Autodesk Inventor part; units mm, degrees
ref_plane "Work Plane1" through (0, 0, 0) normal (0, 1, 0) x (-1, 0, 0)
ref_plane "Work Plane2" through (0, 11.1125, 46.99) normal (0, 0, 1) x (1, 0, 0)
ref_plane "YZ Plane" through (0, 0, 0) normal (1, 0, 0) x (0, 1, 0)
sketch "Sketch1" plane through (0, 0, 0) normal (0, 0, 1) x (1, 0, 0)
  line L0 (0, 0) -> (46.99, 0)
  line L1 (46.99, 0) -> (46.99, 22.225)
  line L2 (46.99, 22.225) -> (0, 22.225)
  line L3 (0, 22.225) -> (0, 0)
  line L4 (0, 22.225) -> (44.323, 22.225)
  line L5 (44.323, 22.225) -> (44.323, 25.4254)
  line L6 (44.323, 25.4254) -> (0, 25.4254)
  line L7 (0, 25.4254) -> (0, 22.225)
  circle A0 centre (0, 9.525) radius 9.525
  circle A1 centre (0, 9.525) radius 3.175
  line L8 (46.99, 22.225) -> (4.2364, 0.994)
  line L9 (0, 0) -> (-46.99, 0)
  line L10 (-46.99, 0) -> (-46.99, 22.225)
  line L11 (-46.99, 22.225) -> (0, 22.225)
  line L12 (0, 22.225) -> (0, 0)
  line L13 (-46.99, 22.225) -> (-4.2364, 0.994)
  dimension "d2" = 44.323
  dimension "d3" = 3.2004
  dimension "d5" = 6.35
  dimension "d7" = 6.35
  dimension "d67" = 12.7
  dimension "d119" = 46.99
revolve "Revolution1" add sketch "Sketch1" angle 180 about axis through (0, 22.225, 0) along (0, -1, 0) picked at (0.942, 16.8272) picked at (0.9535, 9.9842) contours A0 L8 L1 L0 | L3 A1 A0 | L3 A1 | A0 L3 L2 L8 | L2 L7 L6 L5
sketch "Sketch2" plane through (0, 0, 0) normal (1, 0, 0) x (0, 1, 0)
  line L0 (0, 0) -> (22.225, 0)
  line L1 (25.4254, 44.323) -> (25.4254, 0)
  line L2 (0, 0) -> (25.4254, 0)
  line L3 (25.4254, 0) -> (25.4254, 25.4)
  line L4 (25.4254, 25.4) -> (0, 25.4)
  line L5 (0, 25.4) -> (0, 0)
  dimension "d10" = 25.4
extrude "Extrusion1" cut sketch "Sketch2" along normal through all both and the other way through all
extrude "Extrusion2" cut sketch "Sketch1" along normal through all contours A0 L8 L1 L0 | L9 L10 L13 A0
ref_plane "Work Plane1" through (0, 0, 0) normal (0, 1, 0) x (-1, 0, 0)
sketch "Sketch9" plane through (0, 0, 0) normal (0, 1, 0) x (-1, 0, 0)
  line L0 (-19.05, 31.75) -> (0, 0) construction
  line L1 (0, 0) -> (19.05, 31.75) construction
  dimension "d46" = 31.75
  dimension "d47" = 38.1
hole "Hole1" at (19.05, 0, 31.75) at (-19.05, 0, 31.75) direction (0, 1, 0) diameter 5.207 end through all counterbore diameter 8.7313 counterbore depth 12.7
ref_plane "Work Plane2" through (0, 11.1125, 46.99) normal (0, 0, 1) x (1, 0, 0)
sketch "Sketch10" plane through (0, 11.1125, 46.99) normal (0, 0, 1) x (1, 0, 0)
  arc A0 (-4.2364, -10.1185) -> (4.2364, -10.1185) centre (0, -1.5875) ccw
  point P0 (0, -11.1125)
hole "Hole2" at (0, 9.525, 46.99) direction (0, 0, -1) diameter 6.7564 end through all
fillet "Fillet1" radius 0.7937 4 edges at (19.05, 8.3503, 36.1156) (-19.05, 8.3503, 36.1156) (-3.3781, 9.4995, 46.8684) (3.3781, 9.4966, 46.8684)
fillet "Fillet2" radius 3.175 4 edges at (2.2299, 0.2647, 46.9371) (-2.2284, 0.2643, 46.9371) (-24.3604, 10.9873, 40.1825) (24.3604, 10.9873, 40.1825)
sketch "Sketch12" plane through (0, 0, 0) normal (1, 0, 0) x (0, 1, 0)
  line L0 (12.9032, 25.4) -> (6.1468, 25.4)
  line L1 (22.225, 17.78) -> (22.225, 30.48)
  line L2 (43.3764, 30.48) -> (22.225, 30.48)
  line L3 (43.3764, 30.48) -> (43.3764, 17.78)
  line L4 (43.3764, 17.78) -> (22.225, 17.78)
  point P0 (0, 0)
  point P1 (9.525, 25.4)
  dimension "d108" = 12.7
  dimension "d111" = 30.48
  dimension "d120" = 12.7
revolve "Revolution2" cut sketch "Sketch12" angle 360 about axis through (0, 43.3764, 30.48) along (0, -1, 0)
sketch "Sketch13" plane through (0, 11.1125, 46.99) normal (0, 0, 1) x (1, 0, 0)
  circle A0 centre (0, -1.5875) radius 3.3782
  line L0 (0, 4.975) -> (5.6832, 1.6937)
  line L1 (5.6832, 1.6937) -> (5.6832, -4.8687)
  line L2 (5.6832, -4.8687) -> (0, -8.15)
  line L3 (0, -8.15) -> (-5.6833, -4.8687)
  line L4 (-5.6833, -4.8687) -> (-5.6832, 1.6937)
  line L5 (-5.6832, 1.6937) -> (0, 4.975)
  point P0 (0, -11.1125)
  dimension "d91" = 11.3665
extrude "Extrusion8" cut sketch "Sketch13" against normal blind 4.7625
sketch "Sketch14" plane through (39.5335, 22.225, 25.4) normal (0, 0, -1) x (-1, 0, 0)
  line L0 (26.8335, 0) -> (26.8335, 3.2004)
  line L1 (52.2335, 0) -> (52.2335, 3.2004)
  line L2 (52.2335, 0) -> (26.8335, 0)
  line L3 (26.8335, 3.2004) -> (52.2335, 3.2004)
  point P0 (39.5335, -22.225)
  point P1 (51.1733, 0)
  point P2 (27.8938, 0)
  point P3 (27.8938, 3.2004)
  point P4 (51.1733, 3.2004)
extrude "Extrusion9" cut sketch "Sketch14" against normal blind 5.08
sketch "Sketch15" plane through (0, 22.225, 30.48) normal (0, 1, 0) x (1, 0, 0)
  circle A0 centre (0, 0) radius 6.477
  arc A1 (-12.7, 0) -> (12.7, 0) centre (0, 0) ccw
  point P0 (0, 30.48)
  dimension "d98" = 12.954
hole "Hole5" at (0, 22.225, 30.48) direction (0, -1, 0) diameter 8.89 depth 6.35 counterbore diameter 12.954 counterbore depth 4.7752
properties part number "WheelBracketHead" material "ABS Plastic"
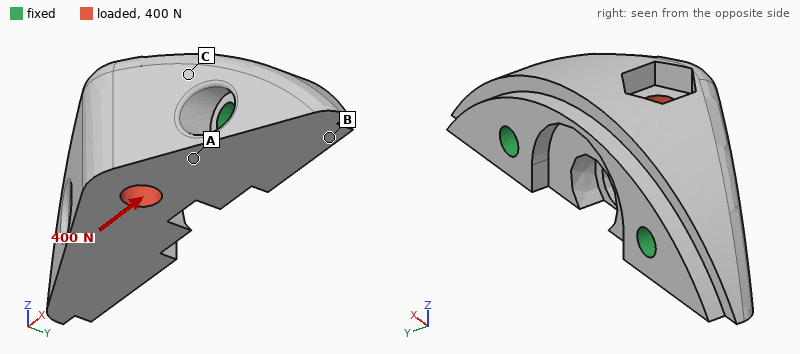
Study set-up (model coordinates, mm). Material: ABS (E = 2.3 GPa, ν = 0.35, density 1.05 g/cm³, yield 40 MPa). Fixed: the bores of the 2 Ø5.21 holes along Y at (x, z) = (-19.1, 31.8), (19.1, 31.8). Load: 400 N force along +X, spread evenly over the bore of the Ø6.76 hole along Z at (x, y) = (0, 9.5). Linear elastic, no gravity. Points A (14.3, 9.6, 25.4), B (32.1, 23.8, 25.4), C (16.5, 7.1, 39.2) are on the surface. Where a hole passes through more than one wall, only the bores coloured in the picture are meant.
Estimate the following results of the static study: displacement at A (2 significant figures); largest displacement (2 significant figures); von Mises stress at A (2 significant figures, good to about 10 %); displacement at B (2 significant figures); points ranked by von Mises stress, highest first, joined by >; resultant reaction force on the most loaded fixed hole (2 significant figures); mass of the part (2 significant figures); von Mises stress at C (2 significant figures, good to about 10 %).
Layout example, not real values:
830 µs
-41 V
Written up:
7.2 µm
16 µm
1.3 MPa
3.3 µm
A > C > B
210 N
19 g
0.73 MPa
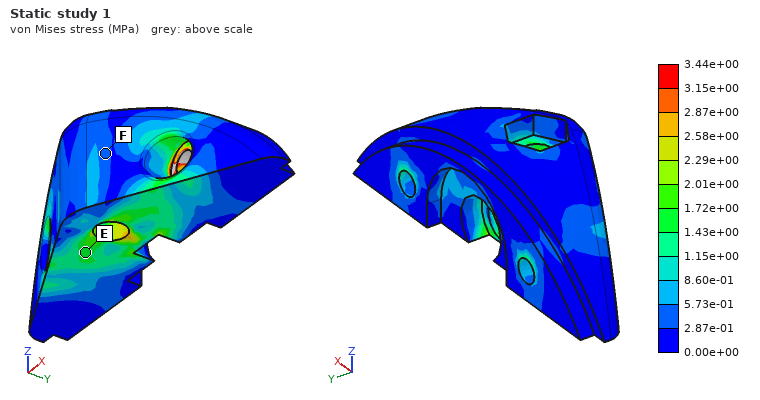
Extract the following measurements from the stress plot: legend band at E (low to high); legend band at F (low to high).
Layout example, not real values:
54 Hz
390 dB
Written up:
1.43e+00 to 1.72e+00 MPa
2.87e-01 to 5.73e-01 MPa
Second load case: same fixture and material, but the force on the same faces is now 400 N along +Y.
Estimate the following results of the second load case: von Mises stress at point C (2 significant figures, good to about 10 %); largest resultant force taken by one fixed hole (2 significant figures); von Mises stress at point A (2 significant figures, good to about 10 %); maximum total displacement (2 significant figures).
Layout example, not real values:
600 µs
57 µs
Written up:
0.62 MPa
230 N
1.1 MPa
25 µm
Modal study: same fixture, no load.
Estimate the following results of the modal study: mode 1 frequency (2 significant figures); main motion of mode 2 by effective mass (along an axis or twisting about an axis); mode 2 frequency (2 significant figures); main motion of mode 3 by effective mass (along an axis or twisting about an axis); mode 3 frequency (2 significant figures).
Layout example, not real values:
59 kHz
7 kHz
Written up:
4800 Hz
along Y
8100 Hz
along X
9500 Hz
